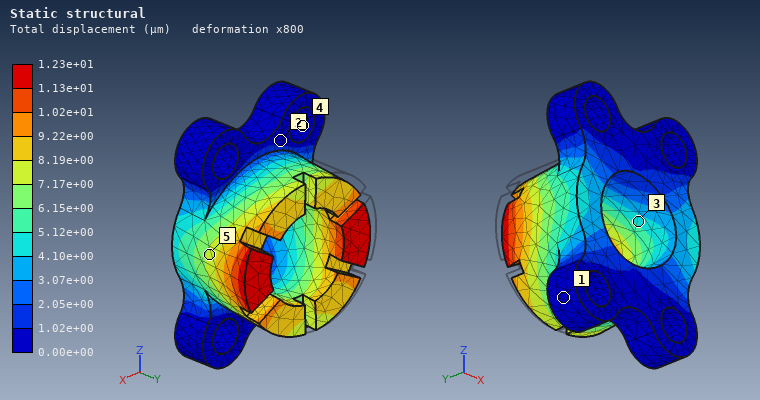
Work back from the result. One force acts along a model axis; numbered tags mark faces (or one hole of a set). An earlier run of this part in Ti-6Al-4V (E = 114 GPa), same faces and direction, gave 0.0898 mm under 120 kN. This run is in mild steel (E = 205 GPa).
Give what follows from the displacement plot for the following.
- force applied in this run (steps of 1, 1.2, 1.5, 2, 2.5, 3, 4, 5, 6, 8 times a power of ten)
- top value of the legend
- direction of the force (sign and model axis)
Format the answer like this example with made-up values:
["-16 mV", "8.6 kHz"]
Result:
["30 kN", "1.23e+01 µm", "+X"]
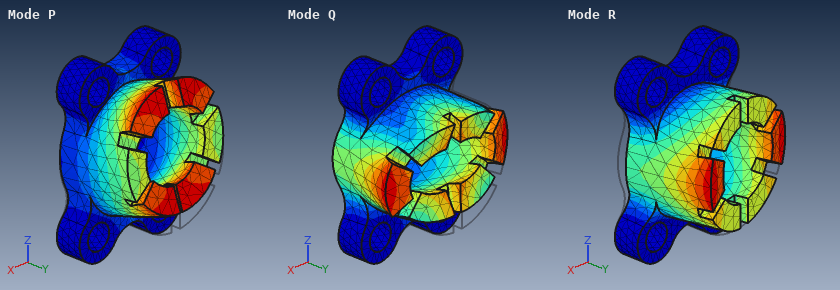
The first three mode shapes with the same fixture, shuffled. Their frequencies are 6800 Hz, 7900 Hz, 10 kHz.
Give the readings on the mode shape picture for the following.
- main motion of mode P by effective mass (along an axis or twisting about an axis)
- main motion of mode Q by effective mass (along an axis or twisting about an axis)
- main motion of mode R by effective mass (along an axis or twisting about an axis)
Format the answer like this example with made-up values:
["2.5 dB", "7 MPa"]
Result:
["along Z", "along Y", "along X"]
